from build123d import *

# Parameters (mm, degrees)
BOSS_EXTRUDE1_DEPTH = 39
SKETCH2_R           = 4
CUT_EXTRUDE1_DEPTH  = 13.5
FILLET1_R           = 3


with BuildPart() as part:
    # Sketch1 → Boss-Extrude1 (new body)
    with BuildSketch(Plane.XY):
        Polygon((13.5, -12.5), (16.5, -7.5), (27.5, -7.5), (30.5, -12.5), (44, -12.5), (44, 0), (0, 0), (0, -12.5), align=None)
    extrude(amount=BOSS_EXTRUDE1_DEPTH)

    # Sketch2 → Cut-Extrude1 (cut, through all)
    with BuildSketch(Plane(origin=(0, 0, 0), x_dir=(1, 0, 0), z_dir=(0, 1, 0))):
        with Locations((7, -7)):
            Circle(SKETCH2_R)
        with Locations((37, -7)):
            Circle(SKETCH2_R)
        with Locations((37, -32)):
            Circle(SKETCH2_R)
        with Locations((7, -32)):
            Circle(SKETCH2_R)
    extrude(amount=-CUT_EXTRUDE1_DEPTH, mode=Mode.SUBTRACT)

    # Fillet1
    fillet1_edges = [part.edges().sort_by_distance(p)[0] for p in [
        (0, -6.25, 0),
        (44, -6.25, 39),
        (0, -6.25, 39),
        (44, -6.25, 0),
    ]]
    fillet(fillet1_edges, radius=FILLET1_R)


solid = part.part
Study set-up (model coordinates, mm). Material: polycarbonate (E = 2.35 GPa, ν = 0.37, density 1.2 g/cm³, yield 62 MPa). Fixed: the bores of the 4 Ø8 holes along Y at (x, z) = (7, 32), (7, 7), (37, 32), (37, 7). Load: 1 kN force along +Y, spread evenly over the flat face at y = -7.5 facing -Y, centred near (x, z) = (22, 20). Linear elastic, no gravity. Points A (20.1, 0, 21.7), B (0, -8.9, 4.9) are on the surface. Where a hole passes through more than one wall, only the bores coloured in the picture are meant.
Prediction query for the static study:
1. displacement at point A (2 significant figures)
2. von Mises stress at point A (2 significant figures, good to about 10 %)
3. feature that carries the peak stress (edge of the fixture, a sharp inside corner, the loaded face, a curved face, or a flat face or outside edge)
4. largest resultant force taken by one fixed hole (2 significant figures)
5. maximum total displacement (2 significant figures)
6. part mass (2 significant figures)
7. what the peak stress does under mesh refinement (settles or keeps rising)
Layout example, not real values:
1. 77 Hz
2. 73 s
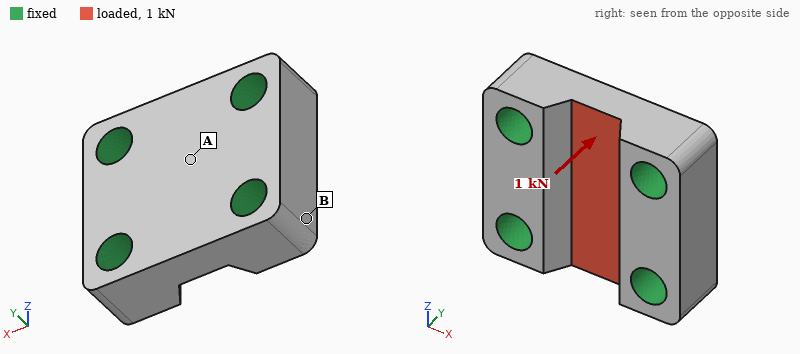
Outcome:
1. 28 µm
2. 3.8 MPa
3. edge of the fixture
4. 260 N
5. 33 µm
6. 19 g
7. keeps rising
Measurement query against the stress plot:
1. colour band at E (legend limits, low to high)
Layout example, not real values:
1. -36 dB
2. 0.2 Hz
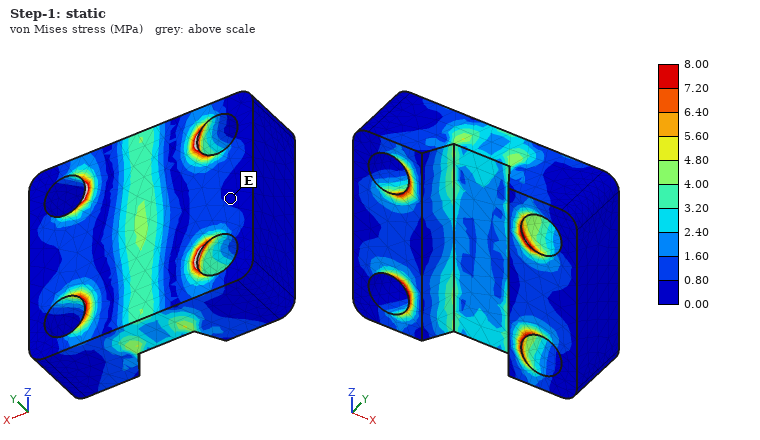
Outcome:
1. 0.00 to 0.80 MPa
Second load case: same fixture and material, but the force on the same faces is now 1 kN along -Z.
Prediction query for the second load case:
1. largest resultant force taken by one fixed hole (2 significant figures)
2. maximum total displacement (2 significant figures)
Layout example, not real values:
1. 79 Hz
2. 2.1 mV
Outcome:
1. 260 N
2. 41 µm
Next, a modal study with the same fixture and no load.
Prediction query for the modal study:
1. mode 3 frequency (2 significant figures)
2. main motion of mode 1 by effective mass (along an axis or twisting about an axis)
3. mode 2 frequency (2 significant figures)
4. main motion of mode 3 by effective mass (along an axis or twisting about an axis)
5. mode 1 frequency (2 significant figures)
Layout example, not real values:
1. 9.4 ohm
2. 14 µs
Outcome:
1. 17 kHz
2. along Y
3. 16 kHz
4. along Z
5. 13 kHz
